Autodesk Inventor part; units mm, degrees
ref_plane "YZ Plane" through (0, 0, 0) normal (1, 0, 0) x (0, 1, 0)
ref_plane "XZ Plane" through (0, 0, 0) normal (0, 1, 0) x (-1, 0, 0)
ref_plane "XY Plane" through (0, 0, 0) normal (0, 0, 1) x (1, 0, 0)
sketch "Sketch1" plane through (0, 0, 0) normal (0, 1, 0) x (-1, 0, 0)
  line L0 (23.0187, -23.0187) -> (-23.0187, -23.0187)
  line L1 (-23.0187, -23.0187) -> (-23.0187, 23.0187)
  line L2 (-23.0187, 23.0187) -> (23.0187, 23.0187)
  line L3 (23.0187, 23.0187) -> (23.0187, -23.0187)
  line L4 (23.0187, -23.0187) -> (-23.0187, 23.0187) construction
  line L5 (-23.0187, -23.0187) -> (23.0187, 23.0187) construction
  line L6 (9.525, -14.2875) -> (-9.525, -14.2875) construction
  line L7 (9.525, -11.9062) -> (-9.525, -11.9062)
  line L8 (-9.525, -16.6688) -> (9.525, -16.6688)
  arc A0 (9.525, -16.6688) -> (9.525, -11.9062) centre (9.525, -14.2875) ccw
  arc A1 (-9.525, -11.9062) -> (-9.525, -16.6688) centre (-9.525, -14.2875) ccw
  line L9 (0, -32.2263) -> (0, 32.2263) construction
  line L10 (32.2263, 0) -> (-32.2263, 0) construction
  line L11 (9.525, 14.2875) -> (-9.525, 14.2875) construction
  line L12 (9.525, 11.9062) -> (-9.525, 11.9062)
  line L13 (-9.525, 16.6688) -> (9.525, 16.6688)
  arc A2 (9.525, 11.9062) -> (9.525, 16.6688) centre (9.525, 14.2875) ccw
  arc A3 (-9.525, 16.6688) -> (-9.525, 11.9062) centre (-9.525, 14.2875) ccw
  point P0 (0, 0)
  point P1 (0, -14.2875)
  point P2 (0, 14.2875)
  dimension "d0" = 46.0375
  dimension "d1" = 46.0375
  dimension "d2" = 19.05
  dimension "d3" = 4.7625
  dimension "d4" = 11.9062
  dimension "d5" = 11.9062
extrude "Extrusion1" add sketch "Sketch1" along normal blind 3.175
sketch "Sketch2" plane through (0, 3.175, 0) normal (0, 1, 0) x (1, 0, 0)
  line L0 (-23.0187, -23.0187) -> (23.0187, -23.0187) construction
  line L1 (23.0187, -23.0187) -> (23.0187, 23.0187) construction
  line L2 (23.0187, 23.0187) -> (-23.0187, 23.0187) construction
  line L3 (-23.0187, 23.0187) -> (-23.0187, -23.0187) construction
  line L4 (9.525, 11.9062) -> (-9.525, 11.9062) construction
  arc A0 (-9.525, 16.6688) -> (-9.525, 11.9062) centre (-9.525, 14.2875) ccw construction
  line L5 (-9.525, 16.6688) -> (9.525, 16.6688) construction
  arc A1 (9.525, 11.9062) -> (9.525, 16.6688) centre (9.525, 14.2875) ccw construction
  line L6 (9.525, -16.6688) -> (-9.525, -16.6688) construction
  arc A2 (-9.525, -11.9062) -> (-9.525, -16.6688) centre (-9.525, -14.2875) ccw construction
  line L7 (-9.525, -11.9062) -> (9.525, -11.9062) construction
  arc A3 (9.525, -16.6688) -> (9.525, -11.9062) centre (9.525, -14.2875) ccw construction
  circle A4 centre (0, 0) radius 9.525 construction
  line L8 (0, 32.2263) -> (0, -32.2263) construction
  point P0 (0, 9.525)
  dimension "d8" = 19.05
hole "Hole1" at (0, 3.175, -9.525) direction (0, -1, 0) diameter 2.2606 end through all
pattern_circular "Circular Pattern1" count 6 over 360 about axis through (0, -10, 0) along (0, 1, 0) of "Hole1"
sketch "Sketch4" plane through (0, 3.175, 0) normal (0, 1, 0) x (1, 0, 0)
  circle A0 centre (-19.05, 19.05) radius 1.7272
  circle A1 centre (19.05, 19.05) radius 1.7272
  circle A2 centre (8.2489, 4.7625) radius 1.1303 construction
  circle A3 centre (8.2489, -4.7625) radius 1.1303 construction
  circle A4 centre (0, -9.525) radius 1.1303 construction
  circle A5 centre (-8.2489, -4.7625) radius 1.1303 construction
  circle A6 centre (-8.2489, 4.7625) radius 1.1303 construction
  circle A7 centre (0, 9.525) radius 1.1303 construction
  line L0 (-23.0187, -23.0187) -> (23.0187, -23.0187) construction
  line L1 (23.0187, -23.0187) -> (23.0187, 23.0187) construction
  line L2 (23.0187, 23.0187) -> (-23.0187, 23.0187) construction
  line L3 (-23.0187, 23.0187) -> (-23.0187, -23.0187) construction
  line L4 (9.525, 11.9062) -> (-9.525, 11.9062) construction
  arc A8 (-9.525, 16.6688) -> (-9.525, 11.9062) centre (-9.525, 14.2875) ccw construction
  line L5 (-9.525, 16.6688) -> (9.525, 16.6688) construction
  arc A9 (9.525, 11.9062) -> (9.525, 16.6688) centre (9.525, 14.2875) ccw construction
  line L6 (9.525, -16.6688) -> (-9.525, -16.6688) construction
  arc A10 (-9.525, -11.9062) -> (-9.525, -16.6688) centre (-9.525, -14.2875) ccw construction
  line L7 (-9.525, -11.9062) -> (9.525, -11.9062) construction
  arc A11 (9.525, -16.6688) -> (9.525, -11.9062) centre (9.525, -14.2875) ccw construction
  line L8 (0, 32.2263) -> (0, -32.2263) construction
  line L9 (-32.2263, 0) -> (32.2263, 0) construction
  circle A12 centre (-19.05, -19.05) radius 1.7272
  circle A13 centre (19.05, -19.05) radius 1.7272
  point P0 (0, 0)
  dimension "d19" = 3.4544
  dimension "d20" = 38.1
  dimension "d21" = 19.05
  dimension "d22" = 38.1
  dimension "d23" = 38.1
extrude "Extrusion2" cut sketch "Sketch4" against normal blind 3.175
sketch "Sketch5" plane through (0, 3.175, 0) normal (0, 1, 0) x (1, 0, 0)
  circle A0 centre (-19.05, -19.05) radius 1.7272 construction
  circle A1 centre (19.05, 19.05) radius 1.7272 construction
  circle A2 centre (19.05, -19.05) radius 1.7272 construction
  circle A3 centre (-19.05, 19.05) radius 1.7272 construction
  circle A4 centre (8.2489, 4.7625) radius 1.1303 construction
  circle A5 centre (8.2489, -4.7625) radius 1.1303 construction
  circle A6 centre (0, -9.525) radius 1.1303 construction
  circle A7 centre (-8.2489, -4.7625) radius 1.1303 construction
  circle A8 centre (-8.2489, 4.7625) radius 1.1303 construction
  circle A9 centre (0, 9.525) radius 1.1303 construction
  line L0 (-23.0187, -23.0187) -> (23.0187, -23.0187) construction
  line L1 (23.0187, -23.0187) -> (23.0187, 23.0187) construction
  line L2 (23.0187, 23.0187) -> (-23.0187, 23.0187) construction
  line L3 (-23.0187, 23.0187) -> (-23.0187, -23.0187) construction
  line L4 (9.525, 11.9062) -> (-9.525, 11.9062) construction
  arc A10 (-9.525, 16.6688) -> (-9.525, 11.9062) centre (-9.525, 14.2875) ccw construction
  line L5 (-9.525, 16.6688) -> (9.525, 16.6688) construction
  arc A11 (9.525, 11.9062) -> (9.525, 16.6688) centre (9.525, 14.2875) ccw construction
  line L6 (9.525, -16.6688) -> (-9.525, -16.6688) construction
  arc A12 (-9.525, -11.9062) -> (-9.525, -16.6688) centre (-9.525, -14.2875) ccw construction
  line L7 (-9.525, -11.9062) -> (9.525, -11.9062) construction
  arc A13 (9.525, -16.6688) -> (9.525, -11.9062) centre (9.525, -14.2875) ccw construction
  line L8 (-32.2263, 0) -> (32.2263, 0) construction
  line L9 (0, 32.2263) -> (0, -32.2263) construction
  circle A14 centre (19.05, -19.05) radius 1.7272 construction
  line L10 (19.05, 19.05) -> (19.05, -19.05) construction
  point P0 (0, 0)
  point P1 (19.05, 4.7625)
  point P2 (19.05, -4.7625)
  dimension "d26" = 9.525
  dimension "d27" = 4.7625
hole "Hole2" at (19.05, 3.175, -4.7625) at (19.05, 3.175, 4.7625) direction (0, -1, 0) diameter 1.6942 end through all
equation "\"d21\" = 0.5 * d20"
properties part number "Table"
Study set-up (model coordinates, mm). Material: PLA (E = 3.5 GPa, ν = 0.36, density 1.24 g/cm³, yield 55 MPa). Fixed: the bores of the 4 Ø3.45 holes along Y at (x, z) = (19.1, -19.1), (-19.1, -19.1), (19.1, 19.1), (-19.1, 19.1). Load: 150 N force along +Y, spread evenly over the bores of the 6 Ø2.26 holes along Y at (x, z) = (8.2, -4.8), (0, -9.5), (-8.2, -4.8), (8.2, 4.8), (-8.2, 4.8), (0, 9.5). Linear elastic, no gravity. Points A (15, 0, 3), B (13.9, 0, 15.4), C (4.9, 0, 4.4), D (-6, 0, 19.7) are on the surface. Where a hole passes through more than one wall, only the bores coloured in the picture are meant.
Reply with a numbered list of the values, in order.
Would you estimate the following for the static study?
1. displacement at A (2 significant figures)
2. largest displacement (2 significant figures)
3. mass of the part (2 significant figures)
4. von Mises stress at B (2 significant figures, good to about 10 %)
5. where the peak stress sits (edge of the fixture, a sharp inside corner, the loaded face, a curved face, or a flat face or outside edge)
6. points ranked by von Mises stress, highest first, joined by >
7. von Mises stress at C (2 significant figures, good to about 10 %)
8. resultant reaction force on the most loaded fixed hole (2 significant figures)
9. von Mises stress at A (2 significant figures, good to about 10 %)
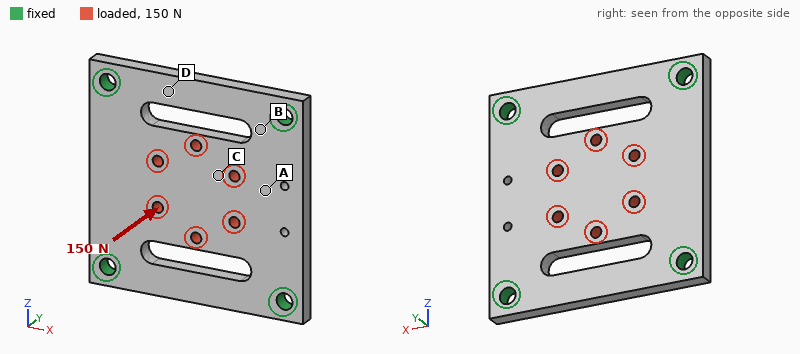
1. 0.14 mm
2. 0.29 mm
3. 7.2 g
4. 11 MPa
5. the loaded face
6. B > C > A > D
7. 8.0 MPa
8. 38 N
9. 5.6 MPa
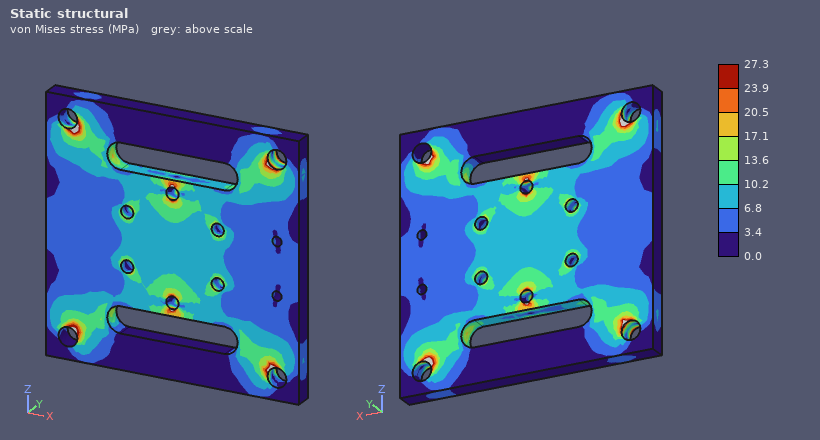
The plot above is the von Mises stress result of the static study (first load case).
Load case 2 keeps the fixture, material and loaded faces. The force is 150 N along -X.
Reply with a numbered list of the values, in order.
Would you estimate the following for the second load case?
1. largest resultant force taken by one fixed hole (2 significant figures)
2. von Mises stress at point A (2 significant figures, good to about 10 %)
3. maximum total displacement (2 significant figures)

1. 44 N
2. 0.42 MPa
3. 15 µm
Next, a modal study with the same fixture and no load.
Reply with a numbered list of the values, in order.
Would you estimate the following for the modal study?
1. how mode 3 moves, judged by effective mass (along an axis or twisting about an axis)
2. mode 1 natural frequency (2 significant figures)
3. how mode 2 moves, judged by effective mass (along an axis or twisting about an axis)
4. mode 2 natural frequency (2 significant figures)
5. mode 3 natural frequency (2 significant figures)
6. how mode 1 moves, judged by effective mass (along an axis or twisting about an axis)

1. twisting about X
2. 2400 Hz
3. twisting about Z
4. 4100 Hz
5. 4400 Hz
6. along Y
